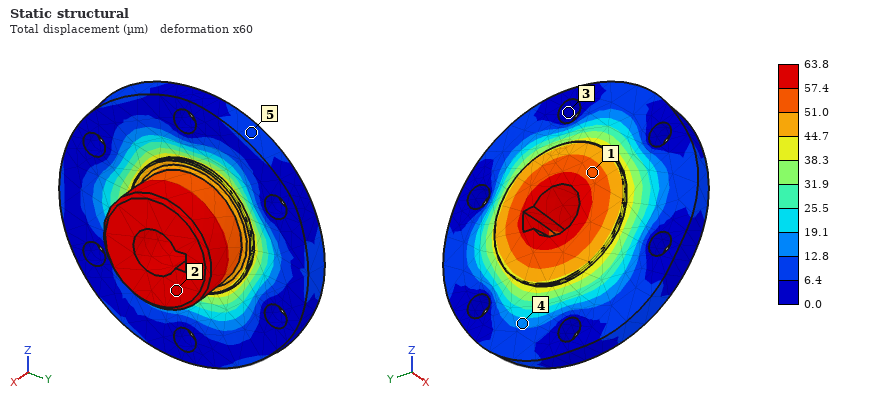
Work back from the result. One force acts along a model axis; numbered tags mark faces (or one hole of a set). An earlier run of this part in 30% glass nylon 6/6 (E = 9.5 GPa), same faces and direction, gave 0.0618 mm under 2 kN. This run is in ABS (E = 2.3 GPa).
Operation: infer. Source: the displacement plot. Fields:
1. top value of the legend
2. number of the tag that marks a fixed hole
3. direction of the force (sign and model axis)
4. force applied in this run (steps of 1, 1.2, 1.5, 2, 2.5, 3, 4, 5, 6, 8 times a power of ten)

63.8 µm
3
-X
500 N
